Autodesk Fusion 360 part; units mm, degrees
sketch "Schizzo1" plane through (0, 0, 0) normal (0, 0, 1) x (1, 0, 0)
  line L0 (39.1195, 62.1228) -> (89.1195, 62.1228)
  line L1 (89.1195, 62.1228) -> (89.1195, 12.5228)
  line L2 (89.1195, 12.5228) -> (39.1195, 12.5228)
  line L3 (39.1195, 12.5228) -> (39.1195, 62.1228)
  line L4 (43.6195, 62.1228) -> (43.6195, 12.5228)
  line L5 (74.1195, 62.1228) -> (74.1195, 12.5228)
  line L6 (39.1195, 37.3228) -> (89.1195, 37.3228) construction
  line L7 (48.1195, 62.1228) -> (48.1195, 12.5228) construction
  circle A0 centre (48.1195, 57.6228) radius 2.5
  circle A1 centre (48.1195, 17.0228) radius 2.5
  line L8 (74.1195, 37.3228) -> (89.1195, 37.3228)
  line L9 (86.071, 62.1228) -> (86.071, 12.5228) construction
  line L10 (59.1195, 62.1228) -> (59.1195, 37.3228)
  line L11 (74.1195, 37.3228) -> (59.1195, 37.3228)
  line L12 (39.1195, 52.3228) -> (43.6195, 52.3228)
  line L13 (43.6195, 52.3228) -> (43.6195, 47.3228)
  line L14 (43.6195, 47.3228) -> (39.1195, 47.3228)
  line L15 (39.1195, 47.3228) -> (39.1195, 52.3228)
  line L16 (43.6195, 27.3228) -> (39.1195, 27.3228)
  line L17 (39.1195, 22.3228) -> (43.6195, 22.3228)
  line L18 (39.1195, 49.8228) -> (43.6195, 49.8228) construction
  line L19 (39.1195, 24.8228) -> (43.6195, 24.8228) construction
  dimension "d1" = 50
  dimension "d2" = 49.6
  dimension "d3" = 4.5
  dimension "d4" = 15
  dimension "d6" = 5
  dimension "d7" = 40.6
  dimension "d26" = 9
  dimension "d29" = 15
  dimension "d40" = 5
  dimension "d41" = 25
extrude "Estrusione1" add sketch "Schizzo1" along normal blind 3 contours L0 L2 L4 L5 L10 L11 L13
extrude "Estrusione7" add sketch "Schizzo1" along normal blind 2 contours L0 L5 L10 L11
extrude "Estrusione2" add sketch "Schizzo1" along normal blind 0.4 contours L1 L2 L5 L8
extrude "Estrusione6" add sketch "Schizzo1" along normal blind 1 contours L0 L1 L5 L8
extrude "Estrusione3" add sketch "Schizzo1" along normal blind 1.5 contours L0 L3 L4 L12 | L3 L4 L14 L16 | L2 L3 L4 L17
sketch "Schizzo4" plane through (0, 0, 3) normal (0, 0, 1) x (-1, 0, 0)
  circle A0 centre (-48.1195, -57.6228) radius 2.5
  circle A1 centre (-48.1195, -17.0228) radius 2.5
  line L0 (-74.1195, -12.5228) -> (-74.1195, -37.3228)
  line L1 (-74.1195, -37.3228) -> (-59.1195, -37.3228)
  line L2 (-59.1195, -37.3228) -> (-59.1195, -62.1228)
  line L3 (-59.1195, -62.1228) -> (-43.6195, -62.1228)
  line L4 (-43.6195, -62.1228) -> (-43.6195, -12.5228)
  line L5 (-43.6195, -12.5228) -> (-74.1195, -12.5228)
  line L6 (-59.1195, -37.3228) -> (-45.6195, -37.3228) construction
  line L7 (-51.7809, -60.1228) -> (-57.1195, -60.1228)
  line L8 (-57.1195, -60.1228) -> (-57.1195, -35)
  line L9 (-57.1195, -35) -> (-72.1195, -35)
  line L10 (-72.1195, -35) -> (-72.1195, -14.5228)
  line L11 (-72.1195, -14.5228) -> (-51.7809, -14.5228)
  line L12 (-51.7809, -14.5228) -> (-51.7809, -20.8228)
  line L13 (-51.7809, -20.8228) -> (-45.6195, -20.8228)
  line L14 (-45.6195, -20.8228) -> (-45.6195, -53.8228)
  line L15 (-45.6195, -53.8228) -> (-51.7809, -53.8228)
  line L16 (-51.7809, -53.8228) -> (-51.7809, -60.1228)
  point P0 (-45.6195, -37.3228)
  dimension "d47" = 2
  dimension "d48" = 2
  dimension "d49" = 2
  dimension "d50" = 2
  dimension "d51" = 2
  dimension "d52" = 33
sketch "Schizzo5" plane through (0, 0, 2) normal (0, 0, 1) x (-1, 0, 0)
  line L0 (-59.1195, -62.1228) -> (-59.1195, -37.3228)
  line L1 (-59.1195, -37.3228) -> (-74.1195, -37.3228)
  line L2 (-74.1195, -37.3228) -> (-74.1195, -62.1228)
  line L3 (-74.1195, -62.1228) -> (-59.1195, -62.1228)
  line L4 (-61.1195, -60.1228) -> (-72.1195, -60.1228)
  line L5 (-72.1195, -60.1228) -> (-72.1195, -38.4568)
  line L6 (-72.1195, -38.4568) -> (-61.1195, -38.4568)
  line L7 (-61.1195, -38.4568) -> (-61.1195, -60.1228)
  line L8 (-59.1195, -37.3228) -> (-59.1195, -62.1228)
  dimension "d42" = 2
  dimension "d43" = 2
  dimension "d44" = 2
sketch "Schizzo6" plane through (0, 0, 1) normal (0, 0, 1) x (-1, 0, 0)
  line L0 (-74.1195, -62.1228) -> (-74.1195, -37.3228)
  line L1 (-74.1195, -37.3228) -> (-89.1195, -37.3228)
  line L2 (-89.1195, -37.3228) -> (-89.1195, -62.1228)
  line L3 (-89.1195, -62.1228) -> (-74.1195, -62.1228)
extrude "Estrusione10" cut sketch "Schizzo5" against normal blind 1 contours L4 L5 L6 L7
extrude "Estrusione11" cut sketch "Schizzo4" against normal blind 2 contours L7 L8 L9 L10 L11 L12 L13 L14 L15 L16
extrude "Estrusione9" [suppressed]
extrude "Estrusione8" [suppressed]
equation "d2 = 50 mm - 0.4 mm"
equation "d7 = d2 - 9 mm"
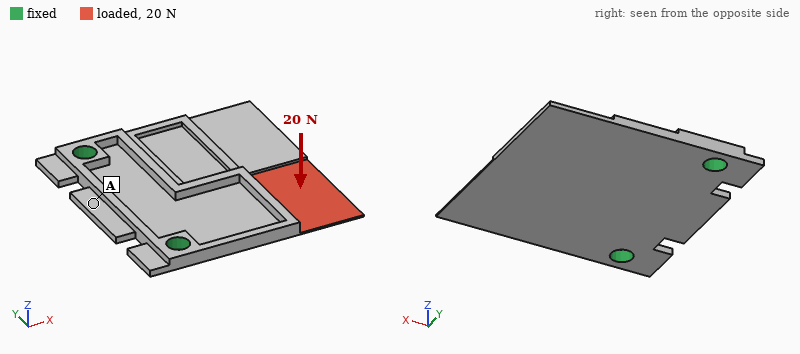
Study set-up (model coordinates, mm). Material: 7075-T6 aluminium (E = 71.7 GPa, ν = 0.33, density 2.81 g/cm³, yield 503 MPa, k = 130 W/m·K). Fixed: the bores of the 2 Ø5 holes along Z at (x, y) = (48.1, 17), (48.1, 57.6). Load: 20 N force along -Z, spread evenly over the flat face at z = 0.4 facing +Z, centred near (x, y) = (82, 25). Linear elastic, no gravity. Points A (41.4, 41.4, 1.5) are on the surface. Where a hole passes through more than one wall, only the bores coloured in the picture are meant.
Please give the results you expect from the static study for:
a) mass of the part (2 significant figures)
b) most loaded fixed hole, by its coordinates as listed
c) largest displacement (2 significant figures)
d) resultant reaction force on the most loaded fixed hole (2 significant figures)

8.7 g
(48.1, 17)
0.85 mm
17 N
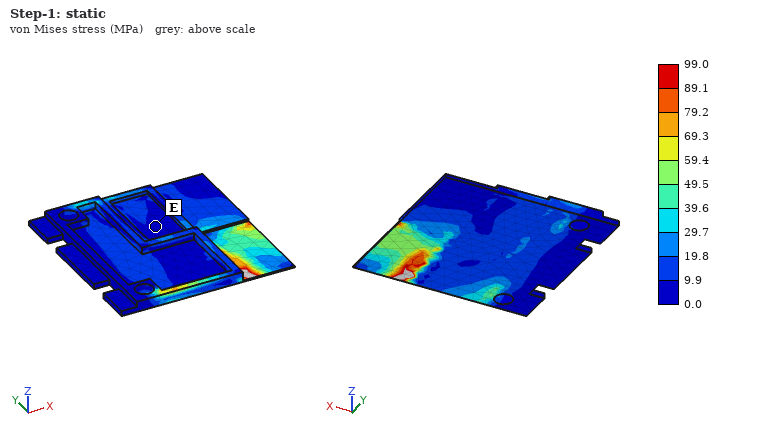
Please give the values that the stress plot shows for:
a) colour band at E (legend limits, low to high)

0.0 to 9.9 MPa
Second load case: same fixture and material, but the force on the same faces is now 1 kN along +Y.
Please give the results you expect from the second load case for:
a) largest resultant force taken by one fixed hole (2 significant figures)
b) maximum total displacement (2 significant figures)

940 N
0.73 mm
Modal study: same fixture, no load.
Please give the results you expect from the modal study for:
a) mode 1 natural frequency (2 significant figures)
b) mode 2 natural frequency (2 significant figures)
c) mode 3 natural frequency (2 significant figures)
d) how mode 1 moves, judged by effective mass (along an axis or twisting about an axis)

1000 Hz
1800 Hz
2800 Hz
along Z
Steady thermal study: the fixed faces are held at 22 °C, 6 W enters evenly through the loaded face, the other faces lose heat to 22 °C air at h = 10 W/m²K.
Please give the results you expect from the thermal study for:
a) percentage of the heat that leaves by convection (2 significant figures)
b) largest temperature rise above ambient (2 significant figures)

11 %
54 K
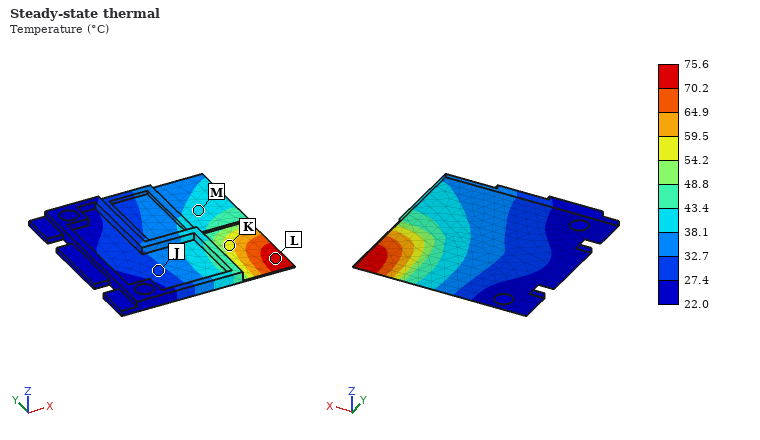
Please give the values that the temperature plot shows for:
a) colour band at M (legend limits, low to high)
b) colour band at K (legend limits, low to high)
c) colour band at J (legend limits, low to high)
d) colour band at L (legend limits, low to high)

38.1 to 43.4 °C
54.2 to 59.5 °C
27.4 to 32.7 °C
70.2 to 75.6 °C
